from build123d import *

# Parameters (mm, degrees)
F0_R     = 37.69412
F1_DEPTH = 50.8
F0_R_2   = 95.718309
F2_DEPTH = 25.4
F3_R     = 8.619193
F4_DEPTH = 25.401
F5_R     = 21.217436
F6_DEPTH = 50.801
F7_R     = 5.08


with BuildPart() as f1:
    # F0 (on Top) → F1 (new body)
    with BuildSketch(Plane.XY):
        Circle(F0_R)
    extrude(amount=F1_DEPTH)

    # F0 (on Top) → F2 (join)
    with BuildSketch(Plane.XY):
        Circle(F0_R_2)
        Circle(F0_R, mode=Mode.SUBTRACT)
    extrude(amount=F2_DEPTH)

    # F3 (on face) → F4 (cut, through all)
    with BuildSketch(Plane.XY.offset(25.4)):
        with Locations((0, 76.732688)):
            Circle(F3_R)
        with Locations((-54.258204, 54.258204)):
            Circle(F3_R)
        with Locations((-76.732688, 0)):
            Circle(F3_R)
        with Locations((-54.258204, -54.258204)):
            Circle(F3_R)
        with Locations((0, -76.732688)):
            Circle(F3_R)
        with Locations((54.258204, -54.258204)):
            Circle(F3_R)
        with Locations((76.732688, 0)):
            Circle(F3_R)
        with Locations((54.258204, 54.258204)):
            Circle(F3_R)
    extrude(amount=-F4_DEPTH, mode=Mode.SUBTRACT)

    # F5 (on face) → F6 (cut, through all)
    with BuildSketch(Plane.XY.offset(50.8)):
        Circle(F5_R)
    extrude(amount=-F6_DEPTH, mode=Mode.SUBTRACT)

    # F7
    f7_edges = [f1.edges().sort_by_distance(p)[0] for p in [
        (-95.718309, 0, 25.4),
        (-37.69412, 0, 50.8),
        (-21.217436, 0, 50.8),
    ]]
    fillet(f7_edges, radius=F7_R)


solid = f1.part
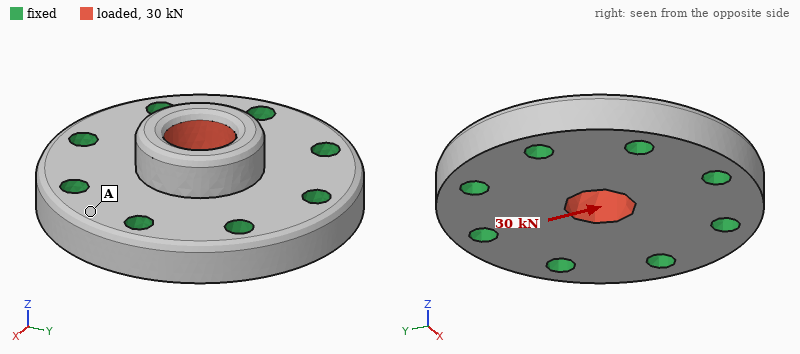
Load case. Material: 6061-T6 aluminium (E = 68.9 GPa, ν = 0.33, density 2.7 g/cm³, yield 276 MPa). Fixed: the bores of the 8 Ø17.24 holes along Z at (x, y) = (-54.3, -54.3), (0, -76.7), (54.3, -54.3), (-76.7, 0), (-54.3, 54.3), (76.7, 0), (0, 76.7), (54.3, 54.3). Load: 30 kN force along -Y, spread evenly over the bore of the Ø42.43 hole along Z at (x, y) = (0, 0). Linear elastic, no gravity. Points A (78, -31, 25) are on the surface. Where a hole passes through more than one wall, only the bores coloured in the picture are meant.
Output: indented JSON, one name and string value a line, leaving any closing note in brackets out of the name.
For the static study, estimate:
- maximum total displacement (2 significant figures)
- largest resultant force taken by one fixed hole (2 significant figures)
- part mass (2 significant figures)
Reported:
{
  "maximum total displacement": "11 µm",
  "largest resultant force taken by one fixed hole": "6.5 kN",
  "part mass": "1.9 kg"
}
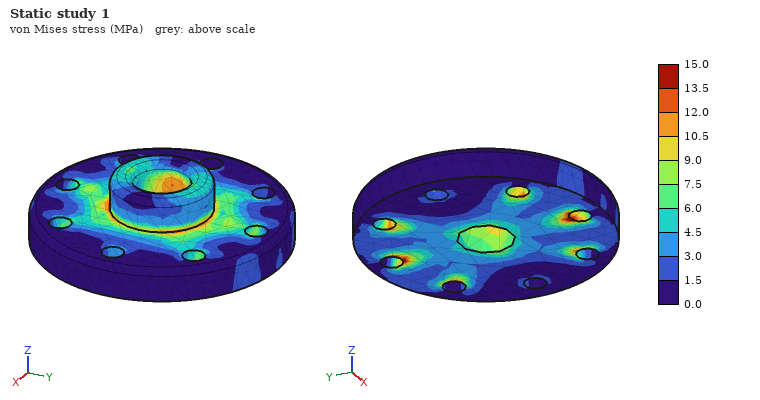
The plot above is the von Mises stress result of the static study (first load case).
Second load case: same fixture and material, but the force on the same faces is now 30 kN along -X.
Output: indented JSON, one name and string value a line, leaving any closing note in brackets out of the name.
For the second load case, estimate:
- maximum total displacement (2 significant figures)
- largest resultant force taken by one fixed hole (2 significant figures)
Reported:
{
  "maximum total displacement": "11 µm",
  "largest resultant force taken by one fixed hole": "6.5 kN"
}
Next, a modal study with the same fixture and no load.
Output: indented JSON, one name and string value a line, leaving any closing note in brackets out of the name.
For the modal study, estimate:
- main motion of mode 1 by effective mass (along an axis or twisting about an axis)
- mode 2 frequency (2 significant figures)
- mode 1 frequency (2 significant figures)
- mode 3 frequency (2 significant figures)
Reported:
{
  "main motion of mode 1 by effective mass": "along Z",
  "mode 2 frequency": "12 kHz",
  "mode 1 frequency": "8800 Hz",
  "mode 3 frequency": "12 kHz"
}
